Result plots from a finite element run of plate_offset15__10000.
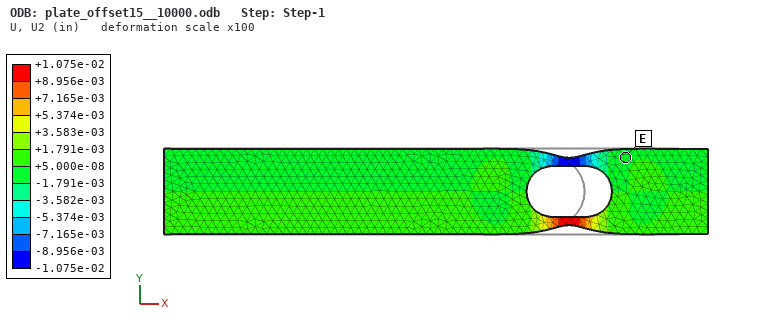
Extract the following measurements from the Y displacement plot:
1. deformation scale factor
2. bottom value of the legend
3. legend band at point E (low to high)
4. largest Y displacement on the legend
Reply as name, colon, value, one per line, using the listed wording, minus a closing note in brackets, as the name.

deformation scale factor: 100
bottom value of the legend: -1.075e-02 in
legend band at point E: -1.791e-03 to +5.000e-08 in
largest Y displacement on the legend: +1.075e-02 in
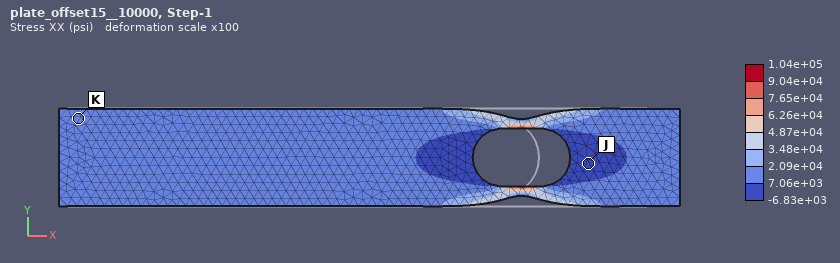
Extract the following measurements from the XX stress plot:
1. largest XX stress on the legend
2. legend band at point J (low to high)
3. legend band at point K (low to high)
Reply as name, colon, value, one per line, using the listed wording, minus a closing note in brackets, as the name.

largest XX stress on the legend: 1.04e+05 psi
legend band at point J: -6.83e+03 to 7.06e+03 psi
legend band at point K: 7.06e+03 to 2.09e+04 psi
